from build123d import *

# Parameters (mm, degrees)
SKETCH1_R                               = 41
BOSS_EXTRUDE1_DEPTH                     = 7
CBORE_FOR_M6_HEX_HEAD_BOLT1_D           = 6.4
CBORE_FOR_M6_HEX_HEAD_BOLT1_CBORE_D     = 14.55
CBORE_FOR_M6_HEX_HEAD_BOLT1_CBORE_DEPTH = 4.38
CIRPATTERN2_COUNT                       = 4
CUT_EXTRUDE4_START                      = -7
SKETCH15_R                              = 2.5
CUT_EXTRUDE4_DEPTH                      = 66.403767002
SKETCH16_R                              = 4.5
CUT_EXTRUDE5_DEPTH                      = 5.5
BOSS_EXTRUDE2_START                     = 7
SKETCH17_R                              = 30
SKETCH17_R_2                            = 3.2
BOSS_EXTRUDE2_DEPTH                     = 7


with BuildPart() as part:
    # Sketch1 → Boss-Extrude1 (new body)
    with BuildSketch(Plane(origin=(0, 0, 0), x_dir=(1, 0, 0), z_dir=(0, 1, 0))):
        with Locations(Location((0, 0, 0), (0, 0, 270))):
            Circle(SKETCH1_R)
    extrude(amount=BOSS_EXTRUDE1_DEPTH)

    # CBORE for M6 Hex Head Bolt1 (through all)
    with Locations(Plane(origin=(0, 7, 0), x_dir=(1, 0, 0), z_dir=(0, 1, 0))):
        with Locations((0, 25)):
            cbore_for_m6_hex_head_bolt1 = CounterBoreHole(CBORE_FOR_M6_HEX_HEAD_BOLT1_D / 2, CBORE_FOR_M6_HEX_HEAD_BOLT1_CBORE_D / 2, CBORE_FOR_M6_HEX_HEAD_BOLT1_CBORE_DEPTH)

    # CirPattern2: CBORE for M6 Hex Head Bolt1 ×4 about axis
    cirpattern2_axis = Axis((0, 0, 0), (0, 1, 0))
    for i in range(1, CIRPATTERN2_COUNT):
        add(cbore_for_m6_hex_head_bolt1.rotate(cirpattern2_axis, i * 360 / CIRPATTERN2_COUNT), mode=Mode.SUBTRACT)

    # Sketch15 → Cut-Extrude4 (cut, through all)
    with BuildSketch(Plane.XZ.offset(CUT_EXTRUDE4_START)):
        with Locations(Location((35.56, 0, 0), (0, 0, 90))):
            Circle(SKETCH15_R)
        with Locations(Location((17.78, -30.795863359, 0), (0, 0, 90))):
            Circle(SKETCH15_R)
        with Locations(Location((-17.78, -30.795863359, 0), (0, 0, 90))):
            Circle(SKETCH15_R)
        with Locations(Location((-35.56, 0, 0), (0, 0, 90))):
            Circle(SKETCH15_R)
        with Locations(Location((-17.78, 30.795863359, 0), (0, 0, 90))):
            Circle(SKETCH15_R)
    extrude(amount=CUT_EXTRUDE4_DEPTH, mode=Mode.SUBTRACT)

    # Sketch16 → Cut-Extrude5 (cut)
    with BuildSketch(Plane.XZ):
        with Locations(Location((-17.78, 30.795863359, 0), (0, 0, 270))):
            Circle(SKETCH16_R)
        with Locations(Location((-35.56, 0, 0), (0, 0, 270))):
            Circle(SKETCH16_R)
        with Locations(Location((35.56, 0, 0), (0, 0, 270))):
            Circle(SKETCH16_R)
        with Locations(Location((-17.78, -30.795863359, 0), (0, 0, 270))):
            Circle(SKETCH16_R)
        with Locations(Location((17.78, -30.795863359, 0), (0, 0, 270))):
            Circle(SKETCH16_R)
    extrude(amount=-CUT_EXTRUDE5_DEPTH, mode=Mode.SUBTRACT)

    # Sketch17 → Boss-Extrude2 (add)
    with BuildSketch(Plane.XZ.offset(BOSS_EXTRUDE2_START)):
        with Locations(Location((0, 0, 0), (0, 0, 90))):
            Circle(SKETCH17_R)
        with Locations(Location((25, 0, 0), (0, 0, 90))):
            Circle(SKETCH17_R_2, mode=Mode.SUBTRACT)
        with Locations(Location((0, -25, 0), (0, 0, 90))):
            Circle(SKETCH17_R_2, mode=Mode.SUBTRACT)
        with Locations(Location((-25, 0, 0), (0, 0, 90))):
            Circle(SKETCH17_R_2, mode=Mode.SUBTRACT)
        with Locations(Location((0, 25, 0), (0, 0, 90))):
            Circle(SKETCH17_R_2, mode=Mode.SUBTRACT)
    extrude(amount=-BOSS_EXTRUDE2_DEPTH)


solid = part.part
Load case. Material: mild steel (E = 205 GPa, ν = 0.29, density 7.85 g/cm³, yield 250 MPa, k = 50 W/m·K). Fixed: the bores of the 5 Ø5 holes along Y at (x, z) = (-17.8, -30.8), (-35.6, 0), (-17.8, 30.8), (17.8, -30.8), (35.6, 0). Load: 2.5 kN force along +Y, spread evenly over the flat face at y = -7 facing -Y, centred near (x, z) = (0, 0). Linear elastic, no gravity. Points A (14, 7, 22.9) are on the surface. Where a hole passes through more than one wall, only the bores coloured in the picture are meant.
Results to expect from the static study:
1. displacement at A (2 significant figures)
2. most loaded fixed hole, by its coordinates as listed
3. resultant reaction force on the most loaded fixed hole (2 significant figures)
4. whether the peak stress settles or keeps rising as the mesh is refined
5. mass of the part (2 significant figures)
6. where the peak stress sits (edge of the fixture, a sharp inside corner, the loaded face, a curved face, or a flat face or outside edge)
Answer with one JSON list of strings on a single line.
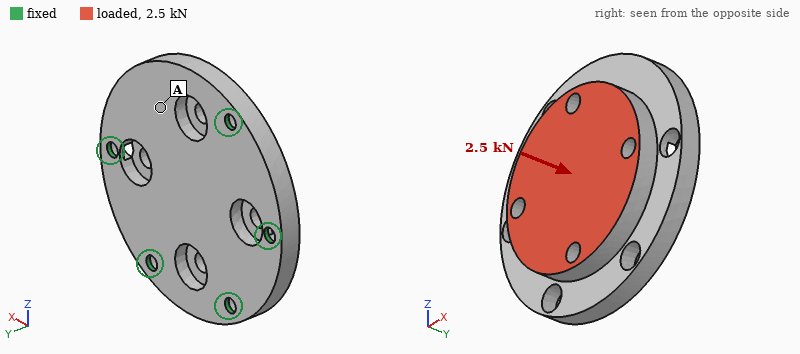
["6.0 µm", "(-17.8, 30.8)", "1.0 kN", "keeps rising", "400 g", "edge of the fixture"]
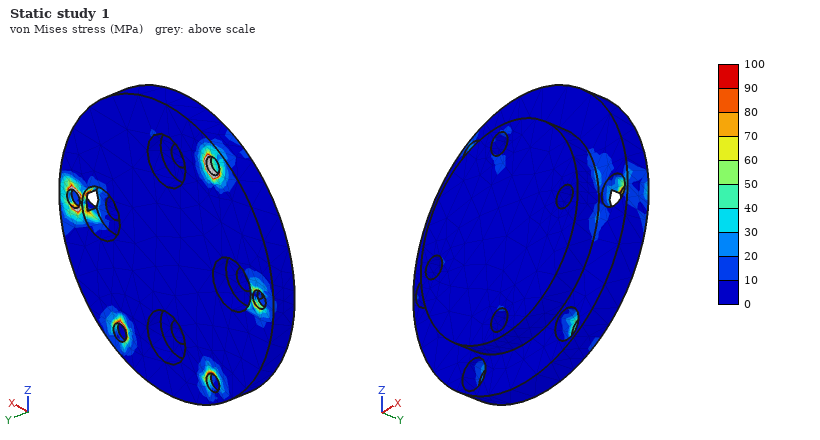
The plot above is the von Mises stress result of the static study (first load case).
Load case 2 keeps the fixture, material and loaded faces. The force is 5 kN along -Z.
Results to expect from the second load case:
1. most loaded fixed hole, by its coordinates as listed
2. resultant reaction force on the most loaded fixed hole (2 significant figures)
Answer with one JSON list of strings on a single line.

["(-17.8, 30.8)", "1.7 kN"]
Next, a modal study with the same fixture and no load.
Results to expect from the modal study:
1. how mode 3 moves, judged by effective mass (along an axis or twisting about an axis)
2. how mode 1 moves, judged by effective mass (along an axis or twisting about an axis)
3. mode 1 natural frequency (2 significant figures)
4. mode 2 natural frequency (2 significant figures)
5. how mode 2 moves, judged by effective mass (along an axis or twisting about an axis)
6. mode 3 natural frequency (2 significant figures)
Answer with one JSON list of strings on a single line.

["along X", "along Y", "5900 Hz", "10000 Hz", "along Y", "12 kHz"]
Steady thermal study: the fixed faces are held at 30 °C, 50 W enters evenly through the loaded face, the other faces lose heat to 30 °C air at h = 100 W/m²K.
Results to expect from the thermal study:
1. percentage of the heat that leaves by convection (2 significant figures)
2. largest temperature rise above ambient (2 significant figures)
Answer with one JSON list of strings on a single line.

["43 %", "27 K"]
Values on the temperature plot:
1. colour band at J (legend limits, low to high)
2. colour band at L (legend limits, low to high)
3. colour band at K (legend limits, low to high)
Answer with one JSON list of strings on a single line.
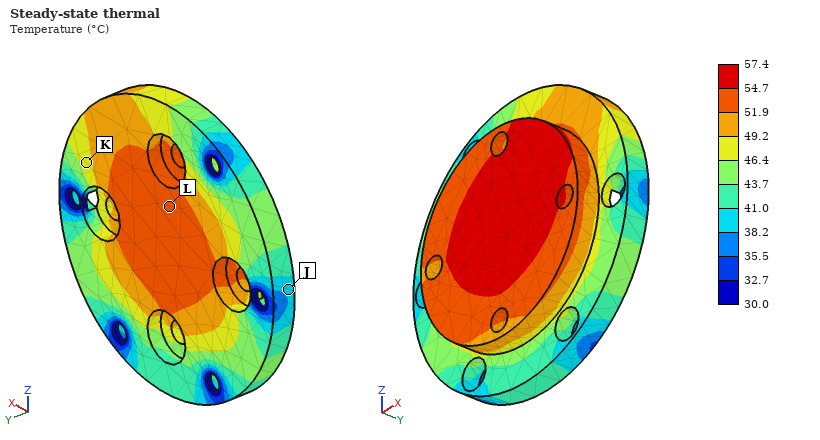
["38.2 to 41.0 °C", "51.9 to 54.7 °C", "46.4 to 49.2 °C"]
